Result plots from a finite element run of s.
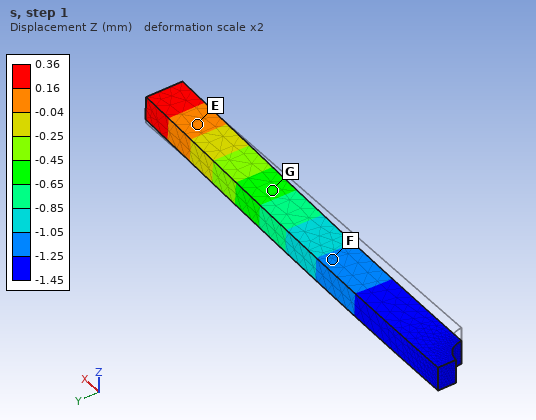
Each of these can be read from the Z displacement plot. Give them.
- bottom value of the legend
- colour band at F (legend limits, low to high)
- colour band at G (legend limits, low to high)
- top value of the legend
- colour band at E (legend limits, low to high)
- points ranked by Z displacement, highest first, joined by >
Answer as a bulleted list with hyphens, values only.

- -1.45 mm
- -1.25 to -1.05 mm
- -0.65 to -0.45 mm
- 0.36 mm
- -0.04 to 0.16 mm
- E > G > F
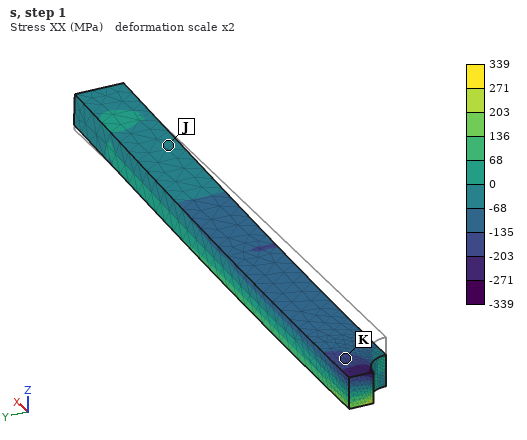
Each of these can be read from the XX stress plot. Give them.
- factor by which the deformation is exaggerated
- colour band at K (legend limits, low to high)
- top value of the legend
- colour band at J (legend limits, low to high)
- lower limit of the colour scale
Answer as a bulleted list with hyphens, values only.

- 2
- -203 to -135 MPa
- 339 MPa
- -68 to 0 MPa
- -339 MPa
